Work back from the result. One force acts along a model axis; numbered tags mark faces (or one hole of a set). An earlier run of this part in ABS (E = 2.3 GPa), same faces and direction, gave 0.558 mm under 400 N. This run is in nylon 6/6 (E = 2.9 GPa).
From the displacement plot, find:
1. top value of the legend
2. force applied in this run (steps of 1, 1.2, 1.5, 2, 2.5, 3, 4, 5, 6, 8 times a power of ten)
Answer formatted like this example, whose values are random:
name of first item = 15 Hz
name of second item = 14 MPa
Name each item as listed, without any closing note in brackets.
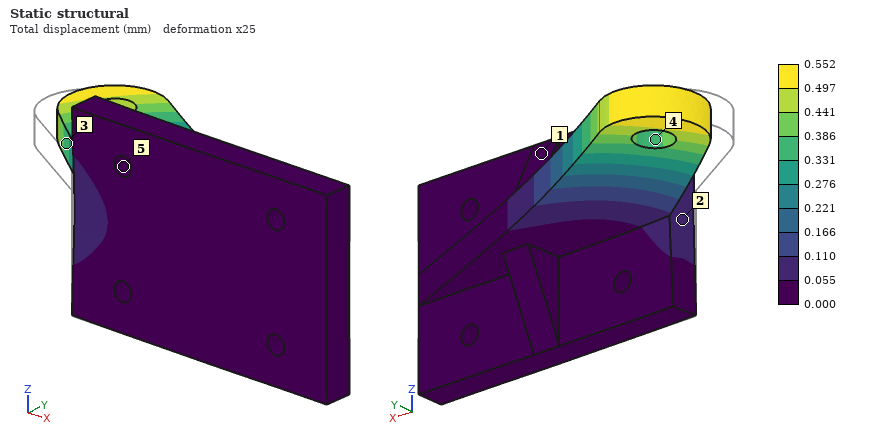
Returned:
top value of the legend = 0.552 mm
force applied in this run = 500 N
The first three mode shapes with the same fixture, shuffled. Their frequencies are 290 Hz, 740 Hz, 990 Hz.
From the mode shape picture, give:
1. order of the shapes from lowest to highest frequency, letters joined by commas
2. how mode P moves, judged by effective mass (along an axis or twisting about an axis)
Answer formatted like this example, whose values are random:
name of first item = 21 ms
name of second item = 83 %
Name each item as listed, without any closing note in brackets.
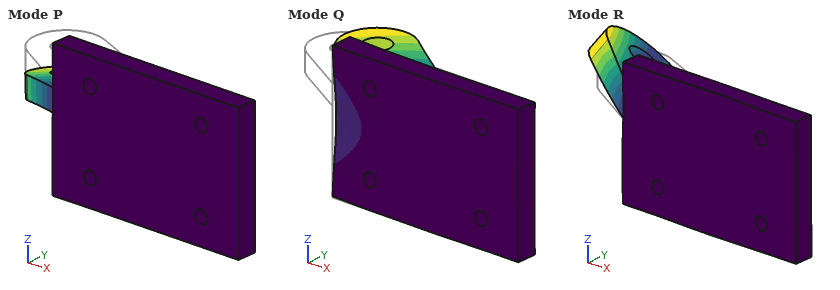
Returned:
order of the shapes from lowest to highest frequency, letters joined by commas = P, Q, R
how mode P moves, judged by effective mass = along Z
